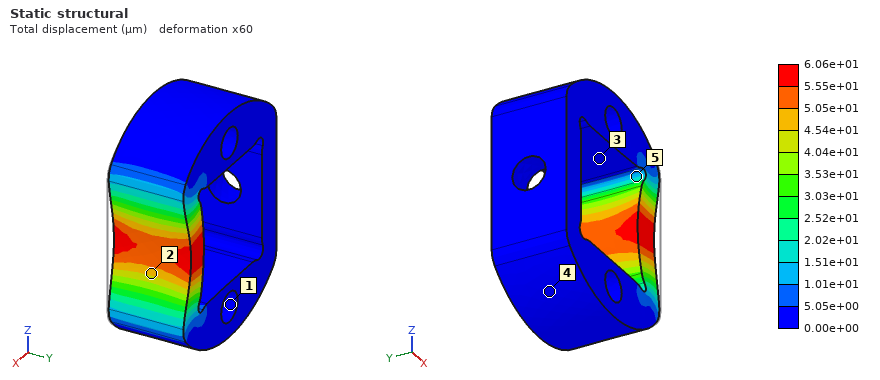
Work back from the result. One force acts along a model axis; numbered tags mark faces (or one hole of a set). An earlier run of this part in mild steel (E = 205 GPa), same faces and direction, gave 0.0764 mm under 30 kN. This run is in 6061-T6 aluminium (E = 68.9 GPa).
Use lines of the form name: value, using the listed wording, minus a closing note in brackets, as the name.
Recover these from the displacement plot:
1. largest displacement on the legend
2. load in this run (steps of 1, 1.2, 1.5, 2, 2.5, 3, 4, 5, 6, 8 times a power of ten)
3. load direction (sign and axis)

largest displacement on the legend: 6.06e+01 µm
load in this run: 8 kN
load direction: -X
